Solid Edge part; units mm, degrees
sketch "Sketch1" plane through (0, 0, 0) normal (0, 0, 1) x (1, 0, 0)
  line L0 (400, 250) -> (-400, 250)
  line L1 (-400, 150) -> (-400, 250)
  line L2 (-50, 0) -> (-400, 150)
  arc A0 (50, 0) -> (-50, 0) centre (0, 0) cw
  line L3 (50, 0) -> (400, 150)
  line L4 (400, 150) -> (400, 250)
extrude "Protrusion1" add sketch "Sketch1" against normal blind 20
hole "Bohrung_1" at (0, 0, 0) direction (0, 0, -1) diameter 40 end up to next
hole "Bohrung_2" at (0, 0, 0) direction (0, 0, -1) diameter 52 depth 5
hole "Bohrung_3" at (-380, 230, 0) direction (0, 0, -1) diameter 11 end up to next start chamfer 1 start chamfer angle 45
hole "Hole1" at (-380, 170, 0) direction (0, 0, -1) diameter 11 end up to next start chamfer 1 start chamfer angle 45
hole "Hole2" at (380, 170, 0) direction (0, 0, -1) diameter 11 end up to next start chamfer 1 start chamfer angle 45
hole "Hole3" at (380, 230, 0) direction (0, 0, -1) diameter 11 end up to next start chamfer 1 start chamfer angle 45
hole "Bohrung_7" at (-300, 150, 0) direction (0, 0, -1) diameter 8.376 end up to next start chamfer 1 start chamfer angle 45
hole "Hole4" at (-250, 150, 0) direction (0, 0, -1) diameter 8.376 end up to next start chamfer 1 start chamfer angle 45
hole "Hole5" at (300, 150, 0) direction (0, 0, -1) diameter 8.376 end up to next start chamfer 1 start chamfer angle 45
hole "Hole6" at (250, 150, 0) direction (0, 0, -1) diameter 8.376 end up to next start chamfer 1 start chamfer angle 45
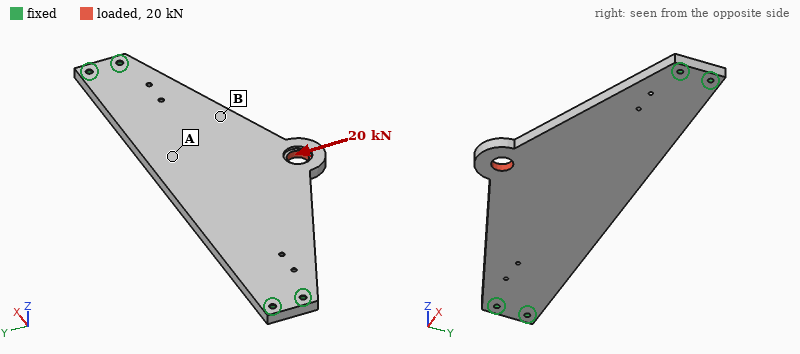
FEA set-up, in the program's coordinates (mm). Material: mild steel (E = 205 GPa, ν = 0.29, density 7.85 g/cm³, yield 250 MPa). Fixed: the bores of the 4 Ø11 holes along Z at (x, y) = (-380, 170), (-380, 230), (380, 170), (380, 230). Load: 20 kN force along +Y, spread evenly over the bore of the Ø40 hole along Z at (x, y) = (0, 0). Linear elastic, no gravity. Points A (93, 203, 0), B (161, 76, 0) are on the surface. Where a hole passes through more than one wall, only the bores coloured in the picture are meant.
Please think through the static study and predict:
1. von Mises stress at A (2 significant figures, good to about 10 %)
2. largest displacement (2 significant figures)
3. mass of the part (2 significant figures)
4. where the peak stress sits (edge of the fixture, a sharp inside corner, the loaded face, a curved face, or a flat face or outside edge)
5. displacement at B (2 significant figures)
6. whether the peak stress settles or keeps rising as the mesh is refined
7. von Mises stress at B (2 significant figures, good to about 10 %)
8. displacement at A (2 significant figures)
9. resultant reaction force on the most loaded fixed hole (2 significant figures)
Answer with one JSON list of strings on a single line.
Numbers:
["3.4 MPa", "89 µm", "23 kg", "edge of the fixture", "33 µm", "keeps rising", "8.8 MPa", "31 µm", "16 kN"]
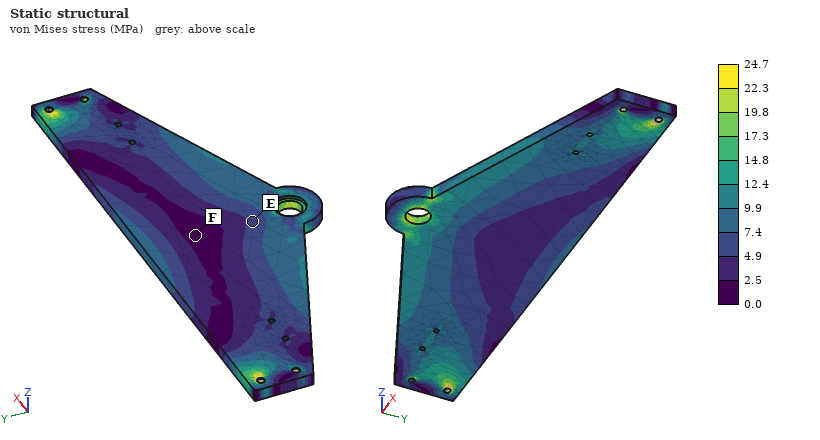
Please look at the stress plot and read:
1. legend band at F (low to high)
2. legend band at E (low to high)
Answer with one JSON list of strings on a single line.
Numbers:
["0.0 to 2.5 MPa", "4.9 to 7.4 MPa"]
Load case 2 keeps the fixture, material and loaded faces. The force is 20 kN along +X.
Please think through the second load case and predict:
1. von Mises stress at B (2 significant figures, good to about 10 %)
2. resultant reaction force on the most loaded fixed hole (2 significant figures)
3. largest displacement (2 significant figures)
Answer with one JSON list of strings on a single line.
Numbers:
["6.0 MPa", "7.0 kN", "25 µm"]
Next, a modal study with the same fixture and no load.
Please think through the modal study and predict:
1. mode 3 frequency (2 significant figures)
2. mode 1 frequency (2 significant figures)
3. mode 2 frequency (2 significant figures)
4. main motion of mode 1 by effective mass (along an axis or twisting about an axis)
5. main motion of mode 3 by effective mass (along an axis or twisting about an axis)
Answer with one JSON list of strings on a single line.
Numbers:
["440 Hz", "140 Hz", "300 Hz", "along Z", "twisting about Y"]
